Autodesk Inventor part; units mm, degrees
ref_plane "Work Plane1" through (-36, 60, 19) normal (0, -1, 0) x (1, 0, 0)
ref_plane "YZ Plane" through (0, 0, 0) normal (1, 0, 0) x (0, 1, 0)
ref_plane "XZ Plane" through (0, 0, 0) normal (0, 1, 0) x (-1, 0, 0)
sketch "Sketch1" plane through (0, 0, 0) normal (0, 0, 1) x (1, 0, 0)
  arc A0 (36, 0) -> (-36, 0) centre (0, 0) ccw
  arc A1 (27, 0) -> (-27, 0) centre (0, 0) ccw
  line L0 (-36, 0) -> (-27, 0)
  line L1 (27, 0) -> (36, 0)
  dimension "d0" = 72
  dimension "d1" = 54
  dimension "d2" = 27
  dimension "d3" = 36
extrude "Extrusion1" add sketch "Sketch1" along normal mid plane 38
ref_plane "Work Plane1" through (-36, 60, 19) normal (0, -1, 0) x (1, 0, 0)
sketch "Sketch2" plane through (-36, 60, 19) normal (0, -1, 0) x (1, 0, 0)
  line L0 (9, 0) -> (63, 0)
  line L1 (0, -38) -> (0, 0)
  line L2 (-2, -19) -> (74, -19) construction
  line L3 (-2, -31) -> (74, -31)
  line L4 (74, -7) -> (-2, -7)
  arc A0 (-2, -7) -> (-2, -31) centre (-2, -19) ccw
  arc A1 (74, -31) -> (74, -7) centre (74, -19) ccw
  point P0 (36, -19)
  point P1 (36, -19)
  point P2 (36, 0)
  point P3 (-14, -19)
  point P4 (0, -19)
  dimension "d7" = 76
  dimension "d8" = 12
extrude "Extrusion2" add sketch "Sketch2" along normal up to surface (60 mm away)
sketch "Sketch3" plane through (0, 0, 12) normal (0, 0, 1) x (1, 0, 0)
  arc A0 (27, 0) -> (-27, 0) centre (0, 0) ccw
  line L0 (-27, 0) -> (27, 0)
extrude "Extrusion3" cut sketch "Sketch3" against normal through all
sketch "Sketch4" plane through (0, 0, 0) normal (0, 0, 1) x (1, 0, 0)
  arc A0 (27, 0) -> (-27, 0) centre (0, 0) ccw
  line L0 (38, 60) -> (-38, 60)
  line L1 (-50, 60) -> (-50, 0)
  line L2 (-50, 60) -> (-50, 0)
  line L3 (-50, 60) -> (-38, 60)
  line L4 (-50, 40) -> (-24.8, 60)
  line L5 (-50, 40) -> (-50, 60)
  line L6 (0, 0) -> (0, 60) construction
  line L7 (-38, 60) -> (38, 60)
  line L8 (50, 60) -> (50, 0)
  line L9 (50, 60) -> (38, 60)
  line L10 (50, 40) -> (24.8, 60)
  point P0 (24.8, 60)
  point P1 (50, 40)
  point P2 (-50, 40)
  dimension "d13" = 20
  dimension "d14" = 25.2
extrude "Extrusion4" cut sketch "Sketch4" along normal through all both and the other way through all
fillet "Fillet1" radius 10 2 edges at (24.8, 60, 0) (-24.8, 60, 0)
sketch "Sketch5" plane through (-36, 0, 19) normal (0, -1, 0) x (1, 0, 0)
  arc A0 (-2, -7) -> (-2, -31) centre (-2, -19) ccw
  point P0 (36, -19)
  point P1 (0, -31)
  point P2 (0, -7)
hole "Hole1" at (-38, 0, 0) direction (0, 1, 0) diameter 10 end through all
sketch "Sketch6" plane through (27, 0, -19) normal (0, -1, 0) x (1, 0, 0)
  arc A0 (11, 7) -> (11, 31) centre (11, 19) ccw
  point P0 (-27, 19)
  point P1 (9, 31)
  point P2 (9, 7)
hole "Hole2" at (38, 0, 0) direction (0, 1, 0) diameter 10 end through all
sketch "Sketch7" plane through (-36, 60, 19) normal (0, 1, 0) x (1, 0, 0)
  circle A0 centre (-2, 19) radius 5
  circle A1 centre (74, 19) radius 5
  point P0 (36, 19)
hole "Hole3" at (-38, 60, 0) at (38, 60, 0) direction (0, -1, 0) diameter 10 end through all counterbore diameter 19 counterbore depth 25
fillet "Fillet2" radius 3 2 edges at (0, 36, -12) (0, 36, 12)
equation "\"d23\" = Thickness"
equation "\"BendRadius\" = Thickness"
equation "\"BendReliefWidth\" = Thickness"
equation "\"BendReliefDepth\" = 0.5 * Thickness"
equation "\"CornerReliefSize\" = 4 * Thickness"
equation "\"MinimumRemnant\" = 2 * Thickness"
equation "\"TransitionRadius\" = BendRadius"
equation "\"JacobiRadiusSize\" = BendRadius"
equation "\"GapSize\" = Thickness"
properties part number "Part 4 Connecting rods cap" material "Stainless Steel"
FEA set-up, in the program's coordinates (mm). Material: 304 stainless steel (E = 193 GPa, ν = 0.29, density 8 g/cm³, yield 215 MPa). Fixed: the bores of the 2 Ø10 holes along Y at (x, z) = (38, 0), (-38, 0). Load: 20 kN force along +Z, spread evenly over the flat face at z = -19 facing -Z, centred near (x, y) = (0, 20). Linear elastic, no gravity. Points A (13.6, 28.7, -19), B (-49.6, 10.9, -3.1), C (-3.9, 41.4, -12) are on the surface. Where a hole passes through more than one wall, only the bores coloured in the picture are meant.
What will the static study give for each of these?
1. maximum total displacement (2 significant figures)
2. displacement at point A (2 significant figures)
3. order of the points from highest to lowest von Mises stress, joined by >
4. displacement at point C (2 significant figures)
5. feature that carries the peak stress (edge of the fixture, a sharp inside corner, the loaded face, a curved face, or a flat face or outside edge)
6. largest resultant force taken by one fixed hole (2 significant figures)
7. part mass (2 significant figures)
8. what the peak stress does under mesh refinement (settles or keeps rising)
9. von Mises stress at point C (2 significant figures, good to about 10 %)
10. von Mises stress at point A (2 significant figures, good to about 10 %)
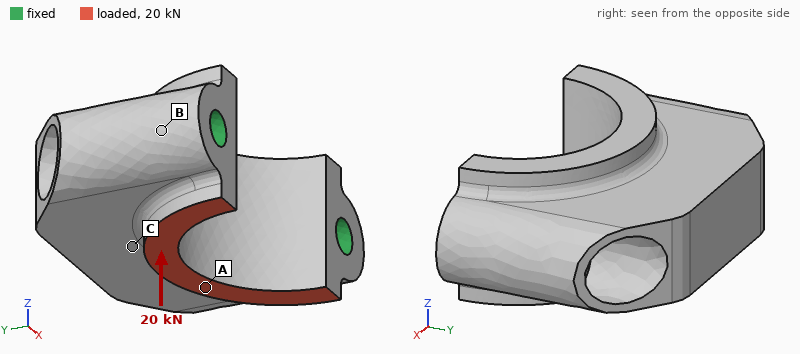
7.3 µm
6.4 µm
A > C > B
6.1 µm
edge of the fixture
10 kN
790 g
keeps rising
12 MPa
24 MPa
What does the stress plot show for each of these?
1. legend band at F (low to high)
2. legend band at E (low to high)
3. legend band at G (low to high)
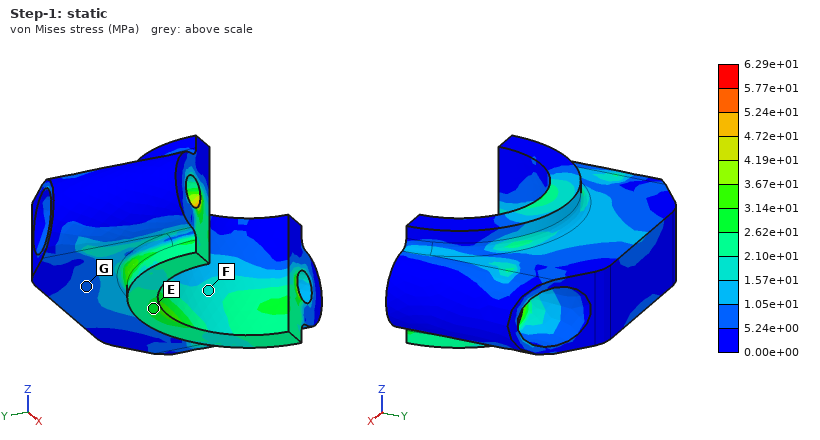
1.57e+01 to 2.10e+01 MPa
2.62e+01 to 3.14e+01 MPa
5.24e+00 to 1.05e+01 MPa
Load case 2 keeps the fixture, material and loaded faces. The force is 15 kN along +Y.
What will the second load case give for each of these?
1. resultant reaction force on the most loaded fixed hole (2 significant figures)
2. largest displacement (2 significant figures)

7.9 kN
14 µm
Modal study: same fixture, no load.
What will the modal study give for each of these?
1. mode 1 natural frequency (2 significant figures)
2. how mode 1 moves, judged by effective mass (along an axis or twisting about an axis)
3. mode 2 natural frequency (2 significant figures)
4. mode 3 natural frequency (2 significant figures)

7700 Hz
along Z
16 kHz
16 kHz
